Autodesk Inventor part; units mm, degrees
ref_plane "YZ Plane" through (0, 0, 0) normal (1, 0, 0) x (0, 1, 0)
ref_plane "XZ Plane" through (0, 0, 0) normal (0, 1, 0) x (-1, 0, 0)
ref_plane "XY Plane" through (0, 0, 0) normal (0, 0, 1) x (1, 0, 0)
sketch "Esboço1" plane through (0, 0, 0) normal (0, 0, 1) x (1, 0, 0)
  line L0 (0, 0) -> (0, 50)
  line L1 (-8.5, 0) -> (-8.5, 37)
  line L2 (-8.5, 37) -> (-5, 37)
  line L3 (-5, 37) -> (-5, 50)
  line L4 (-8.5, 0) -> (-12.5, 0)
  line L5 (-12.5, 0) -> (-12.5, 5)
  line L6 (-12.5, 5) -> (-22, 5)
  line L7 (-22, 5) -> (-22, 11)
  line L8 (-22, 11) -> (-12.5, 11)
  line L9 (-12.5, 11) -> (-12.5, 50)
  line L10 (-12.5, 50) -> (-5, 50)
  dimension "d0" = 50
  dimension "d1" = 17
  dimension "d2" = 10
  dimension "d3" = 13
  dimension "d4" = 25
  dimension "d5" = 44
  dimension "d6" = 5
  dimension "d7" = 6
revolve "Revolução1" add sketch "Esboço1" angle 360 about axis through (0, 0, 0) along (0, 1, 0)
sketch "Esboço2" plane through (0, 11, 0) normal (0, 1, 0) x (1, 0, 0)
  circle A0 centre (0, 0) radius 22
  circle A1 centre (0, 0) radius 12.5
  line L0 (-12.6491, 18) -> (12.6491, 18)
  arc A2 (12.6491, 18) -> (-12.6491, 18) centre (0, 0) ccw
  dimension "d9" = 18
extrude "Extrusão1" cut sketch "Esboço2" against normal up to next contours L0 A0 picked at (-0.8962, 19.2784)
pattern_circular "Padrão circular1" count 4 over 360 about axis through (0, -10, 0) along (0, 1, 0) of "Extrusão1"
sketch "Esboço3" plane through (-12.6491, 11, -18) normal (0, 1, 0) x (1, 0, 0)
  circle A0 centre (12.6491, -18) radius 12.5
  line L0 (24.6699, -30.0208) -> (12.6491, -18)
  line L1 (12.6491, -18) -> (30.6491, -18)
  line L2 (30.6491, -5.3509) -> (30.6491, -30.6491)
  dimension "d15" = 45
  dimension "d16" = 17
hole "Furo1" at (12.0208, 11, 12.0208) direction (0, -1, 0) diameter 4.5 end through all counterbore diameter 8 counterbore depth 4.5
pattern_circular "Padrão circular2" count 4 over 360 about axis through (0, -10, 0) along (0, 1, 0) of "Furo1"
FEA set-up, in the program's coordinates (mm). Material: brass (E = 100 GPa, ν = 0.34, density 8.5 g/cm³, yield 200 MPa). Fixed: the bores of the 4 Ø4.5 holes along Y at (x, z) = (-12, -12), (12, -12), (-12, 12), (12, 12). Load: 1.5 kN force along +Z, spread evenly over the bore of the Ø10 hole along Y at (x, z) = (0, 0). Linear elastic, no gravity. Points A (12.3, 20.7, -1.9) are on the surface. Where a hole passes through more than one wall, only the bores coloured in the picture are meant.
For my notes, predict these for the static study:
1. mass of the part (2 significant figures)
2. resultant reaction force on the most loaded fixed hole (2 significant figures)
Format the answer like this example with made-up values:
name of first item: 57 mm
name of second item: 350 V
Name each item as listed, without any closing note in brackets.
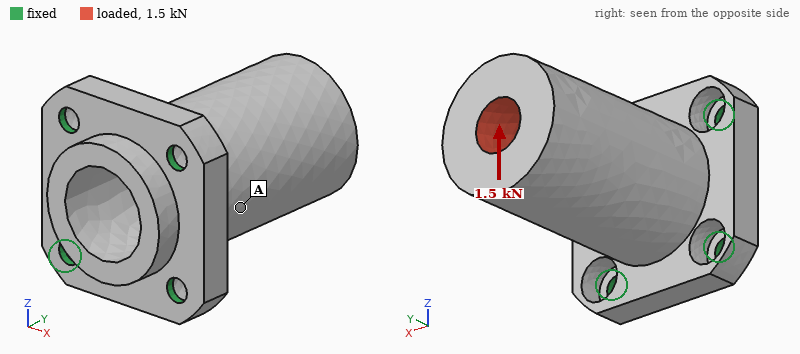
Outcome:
mass of the part: 160 g
resultant reaction force on the most loaded fixed hole: 1.3 kN
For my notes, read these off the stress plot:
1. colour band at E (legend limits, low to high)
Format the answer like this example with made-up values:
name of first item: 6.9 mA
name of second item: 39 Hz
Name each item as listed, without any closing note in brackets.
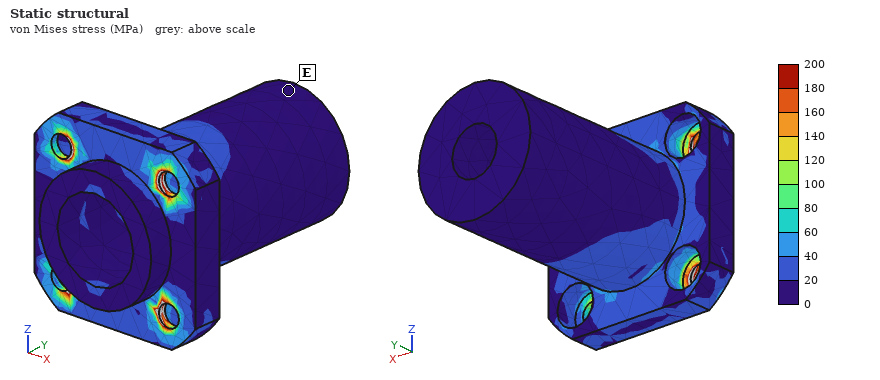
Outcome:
colour band at E: 0 to 20 MPa
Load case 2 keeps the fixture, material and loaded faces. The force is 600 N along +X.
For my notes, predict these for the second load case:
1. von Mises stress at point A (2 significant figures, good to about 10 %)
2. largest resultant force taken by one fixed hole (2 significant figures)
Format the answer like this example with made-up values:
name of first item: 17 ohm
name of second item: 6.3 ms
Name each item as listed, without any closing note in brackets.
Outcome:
von Mises stress at point A: 10 MPa
largest resultant force taken by one fixed hole: 530 N
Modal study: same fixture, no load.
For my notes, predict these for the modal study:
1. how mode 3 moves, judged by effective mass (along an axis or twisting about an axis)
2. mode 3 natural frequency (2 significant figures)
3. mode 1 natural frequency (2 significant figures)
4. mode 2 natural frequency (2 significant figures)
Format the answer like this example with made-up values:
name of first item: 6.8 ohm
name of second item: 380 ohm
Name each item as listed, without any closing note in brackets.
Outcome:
how mode 3 moves, judged by effective mass: along Y
mode 3 natural frequency: 8800 Hz
mode 1 natural frequency: 3400 Hz
mode 2 natural frequency: 3400 Hz
